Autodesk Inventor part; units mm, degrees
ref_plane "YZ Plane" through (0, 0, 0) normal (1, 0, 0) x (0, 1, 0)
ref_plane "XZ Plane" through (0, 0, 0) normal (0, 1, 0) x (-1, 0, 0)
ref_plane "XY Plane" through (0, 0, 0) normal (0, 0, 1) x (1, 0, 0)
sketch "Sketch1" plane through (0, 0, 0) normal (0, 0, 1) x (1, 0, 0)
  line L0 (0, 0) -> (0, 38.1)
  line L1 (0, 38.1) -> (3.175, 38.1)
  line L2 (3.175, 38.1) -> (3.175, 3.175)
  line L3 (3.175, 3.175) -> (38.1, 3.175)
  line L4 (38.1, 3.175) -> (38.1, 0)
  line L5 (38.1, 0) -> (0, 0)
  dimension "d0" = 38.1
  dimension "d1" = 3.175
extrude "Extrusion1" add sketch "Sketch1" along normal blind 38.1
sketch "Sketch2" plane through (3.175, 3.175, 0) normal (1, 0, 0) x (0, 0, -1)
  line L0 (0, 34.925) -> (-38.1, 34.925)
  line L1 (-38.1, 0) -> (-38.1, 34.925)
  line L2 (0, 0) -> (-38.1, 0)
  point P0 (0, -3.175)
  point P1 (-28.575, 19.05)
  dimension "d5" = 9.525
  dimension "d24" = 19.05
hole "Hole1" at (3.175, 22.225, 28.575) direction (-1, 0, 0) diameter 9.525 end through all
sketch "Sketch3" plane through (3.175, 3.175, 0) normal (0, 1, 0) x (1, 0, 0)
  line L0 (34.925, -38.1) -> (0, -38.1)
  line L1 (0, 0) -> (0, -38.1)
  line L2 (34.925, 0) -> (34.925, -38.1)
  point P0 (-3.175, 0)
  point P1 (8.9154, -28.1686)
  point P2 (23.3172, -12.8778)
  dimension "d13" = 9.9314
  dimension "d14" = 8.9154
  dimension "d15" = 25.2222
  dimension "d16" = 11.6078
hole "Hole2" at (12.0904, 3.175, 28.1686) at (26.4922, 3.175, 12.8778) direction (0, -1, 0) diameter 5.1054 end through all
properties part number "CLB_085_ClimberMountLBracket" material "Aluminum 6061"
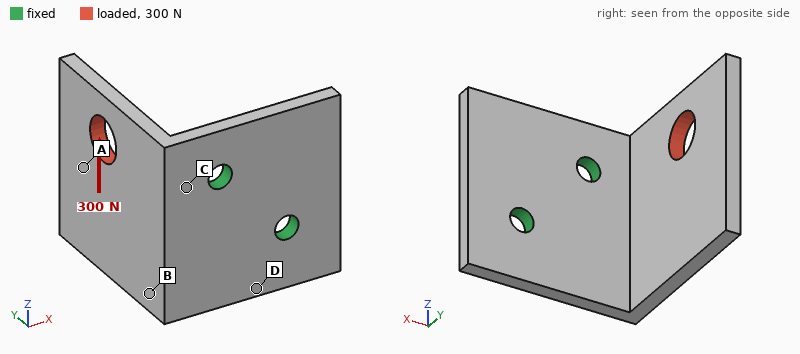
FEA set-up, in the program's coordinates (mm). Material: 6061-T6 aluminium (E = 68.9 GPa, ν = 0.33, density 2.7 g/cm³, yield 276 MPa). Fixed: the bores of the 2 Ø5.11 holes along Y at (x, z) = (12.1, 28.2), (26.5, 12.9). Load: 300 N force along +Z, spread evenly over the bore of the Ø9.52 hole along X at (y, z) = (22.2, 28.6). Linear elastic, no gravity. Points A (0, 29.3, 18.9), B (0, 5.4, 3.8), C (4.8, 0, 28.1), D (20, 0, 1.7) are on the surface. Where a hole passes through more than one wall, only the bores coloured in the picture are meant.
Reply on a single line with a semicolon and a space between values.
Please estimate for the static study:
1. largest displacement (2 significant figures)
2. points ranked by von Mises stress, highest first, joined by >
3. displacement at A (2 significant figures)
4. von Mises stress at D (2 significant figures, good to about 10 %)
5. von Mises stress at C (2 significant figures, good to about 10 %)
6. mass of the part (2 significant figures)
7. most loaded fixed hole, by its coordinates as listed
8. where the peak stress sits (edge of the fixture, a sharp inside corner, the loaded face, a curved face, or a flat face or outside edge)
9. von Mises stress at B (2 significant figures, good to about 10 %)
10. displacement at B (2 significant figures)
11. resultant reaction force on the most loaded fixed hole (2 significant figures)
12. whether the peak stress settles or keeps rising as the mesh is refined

0.24 mm; C > D > B > A; 0.14 mm; 37 MPa; 54 MPa; 23 g; (12.1, 28.2); edge of the fixture; 20 MPa; 0.12 mm; 360 N; keeps rising
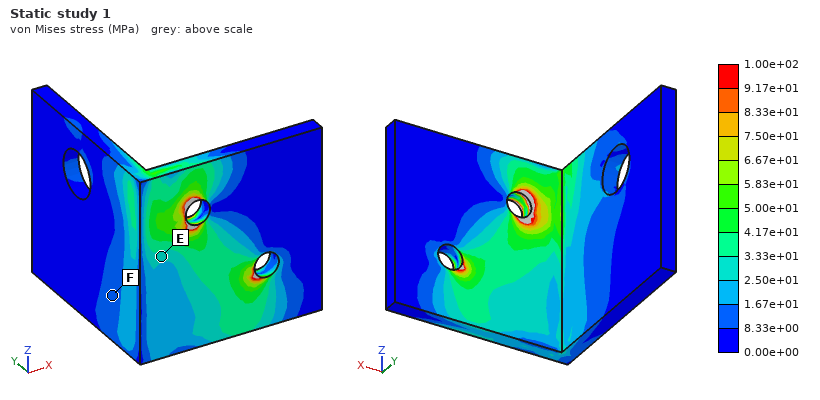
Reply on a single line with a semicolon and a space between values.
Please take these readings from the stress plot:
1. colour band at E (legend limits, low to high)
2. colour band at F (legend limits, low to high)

2.50e+01 to 3.33e+01 MPa; 8.33e+00 to 1.67e+01 MPa
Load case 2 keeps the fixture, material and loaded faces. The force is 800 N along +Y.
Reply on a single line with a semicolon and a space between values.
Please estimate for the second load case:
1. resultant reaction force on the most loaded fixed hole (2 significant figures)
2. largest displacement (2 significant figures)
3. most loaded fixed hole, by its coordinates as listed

880 N; 0.26 mm; (12.1, 28.2)
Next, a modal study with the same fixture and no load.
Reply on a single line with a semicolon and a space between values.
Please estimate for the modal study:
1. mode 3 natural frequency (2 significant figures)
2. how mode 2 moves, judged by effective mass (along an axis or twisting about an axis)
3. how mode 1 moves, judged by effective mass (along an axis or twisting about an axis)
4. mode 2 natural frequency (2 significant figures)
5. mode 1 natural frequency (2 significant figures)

4100 Hz; along Z; along X; 2200 Hz; 1300 Hz
